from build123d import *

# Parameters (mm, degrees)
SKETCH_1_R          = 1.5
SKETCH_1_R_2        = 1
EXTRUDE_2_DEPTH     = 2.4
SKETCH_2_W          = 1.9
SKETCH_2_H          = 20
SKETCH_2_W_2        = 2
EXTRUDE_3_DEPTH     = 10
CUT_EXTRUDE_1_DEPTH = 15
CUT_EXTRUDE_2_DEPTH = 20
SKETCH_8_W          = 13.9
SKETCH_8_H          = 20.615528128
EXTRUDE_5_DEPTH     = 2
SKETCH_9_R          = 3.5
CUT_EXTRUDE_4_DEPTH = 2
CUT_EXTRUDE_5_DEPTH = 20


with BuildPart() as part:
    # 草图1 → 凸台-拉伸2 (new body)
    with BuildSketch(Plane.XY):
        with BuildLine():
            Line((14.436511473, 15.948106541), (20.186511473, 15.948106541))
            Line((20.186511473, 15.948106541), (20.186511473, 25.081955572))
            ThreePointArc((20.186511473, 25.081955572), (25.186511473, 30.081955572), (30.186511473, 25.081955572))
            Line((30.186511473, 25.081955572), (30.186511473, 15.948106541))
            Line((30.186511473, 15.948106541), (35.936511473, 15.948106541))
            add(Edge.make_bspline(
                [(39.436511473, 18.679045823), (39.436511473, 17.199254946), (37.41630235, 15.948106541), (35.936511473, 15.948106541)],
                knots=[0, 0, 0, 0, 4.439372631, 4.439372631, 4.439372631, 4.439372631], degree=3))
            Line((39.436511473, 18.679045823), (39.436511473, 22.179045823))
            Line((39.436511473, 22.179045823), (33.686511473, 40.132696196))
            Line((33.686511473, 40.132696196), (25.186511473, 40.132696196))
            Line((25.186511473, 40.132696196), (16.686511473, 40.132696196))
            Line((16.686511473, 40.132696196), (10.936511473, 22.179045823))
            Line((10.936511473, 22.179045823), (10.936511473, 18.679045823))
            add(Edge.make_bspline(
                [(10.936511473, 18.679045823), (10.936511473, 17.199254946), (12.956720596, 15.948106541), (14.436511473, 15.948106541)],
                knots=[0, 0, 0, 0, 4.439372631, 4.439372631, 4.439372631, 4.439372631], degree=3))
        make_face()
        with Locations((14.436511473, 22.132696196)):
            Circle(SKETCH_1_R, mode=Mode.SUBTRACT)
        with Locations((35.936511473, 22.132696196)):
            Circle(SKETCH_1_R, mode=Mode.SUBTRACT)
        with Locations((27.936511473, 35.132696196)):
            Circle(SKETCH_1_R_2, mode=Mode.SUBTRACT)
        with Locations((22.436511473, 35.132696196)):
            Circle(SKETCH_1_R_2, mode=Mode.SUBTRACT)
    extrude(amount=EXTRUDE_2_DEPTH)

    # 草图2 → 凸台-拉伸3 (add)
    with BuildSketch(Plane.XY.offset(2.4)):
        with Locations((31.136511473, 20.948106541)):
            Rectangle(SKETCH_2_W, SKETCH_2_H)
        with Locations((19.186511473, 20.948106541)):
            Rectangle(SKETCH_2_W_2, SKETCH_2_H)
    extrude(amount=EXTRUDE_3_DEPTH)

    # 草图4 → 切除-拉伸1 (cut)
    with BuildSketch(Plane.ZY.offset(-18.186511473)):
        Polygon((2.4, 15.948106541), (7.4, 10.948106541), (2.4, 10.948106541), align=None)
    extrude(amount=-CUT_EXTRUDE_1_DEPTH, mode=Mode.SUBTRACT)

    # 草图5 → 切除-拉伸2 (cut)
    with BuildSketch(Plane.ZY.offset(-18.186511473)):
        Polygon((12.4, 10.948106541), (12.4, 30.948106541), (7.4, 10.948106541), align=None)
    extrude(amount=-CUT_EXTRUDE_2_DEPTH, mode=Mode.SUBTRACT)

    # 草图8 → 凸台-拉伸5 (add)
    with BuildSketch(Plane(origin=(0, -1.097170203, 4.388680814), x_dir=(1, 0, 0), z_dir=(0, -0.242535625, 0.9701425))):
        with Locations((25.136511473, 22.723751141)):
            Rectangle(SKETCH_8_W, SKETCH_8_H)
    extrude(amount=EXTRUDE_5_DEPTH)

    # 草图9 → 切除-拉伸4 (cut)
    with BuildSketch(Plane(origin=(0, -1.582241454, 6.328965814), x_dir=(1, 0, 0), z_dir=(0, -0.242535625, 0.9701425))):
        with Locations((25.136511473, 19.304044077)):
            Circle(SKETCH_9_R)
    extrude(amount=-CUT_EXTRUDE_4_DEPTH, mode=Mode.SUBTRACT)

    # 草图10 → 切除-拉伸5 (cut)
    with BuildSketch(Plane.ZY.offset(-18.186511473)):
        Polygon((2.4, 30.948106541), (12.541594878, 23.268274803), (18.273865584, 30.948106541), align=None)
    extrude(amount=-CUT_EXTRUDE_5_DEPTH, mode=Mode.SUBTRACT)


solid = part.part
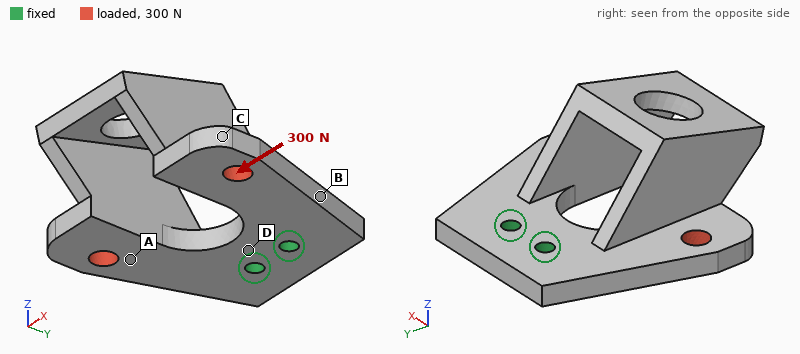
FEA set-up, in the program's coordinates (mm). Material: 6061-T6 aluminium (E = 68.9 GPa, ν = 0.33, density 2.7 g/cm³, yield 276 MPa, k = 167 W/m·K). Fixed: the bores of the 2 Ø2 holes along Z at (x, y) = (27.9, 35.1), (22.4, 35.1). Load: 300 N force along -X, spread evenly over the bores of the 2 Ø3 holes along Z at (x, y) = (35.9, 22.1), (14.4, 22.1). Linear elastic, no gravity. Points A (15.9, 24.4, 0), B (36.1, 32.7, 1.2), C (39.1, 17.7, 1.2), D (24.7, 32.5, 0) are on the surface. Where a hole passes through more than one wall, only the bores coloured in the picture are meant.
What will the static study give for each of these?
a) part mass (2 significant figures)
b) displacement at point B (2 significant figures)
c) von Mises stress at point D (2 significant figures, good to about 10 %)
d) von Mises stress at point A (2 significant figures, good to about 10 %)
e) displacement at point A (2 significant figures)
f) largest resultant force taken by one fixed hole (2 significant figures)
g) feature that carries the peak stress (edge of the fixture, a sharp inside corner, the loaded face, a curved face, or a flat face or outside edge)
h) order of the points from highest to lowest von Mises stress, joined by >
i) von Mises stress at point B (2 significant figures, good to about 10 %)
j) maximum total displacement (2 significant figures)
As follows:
4.7 g
12 µm
65 MPa
23 MPa
23 µm
500 N
edge of the fixture
D > B > A > C
35 MPa
45 µm
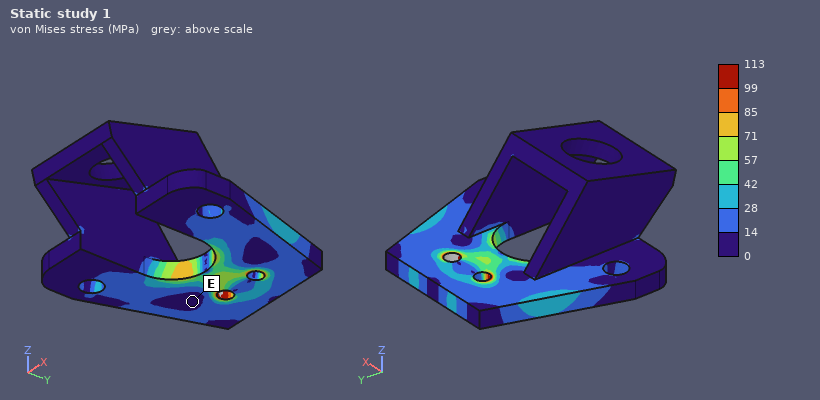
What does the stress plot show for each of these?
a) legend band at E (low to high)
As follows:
0 to 14 MPa
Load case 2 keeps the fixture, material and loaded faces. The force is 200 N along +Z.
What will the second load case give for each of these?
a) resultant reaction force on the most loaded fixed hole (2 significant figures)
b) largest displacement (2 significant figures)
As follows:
100 N
0.24 mm
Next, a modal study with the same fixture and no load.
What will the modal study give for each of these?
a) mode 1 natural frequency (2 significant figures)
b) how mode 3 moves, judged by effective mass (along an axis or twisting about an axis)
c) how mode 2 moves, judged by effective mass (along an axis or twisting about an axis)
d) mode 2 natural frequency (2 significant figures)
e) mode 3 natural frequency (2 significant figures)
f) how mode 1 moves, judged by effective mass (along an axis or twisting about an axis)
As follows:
2900 Hz
along X
along X
5500 Hz
7800 Hz
along Z
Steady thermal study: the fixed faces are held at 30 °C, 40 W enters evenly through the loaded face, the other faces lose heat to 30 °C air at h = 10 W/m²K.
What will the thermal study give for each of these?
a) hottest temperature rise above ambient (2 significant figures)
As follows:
89 K
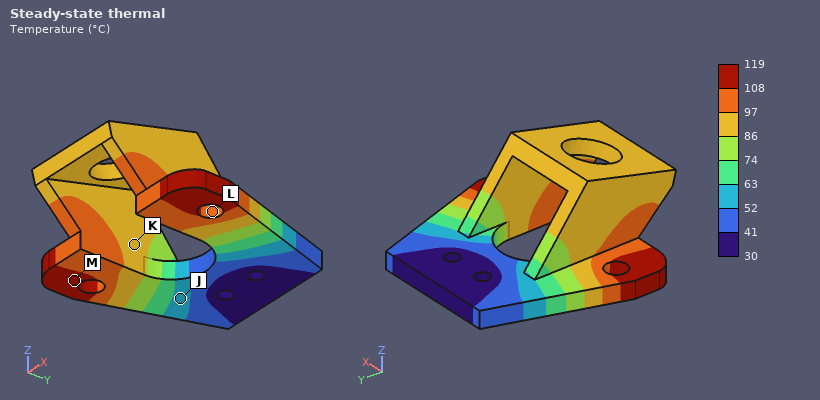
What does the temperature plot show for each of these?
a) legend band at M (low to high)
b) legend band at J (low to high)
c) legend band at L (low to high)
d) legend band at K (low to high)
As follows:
108 to 119 °C
52 to 63 °C
97 to 108 °C
86 to 97 °C
